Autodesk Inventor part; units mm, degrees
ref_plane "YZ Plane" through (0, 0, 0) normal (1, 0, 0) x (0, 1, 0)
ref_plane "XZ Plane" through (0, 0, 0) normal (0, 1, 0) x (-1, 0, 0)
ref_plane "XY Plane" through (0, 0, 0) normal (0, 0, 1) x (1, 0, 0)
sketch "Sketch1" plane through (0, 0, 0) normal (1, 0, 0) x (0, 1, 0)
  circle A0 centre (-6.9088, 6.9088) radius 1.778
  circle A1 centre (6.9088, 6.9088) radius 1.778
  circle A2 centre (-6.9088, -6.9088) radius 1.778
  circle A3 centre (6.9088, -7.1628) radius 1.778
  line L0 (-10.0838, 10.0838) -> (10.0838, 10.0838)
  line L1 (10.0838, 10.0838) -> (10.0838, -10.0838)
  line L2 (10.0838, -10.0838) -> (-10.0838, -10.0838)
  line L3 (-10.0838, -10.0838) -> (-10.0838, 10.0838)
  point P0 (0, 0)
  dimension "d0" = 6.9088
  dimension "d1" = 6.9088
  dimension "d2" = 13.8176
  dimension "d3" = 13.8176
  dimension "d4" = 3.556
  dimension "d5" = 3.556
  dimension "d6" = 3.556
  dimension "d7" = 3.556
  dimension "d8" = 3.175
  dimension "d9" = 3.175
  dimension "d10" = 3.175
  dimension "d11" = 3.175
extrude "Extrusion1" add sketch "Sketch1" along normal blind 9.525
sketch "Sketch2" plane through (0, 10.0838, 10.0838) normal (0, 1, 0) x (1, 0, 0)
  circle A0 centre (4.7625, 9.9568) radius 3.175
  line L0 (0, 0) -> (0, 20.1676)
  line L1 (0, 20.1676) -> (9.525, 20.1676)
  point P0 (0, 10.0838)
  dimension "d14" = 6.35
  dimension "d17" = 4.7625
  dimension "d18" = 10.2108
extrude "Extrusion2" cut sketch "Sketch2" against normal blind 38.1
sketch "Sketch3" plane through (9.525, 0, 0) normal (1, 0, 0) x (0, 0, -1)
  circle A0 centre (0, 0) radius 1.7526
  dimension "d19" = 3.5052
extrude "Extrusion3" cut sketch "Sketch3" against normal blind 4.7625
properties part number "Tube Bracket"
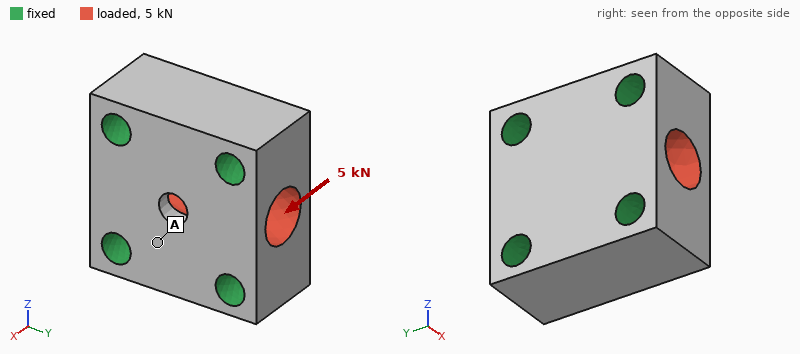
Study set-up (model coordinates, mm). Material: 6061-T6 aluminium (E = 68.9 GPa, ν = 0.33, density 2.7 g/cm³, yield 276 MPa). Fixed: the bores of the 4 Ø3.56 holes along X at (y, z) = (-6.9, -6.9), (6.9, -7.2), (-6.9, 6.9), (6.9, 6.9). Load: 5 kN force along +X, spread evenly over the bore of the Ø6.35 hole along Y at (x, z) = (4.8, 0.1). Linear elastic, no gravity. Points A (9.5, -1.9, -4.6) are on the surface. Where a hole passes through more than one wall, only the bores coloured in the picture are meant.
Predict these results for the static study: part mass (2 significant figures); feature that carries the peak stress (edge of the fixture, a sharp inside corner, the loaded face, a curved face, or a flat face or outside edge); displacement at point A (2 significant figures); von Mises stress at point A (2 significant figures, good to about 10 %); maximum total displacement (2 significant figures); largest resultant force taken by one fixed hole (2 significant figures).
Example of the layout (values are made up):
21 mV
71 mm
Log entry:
7.7 g
a curved face
2.6 µm
8.9 MPa
5.9 µm
1.3 kN
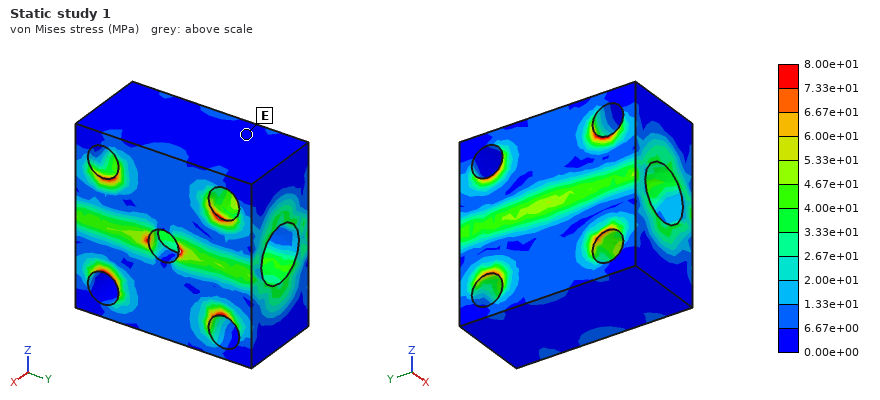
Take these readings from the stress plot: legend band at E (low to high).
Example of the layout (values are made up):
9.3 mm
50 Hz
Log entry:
0.00e+00 to 6.67e+00 MPa
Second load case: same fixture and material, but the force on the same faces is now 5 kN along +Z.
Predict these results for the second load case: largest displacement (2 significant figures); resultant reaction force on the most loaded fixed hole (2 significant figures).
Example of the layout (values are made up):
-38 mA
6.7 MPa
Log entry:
2.1 µm
1.3 kN
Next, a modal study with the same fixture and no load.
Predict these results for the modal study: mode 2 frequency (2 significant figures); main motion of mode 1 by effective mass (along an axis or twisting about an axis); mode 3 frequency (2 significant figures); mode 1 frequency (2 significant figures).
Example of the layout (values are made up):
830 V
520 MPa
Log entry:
110 kHz
along X
120 kHz
100 kHz
